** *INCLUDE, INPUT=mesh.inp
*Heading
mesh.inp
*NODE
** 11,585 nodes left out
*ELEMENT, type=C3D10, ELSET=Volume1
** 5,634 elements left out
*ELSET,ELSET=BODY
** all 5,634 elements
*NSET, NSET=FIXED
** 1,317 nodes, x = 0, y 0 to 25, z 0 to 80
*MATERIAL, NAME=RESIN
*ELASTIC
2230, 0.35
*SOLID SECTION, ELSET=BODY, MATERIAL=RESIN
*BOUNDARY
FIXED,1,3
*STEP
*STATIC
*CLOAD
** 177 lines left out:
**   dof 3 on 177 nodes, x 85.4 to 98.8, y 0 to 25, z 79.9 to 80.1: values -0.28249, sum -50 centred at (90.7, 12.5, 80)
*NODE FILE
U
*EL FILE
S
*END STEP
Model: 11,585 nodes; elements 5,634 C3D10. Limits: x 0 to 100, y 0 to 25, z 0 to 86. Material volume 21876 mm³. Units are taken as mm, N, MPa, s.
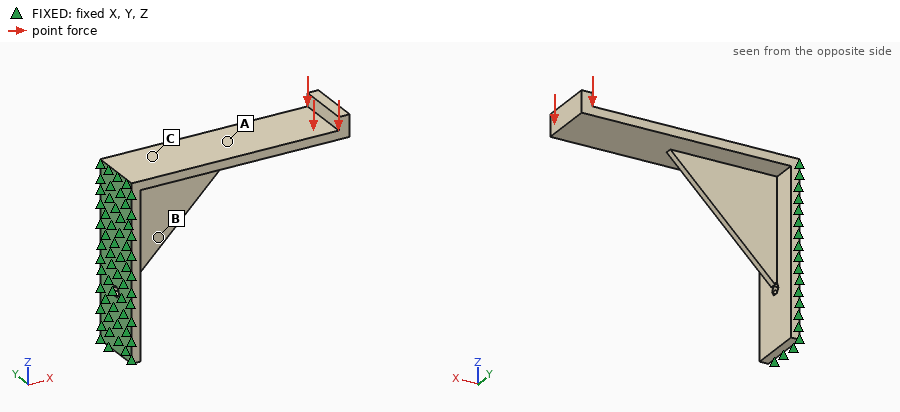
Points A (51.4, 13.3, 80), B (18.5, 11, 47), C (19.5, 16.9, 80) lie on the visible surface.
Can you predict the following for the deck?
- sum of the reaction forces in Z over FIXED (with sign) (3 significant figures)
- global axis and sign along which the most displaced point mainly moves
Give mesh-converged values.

50.0 N
-Z
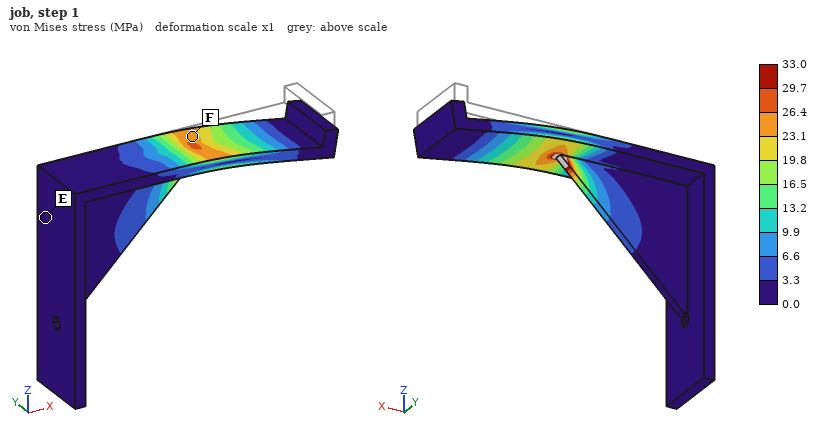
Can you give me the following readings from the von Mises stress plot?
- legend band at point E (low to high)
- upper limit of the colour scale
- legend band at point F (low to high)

0.0 to 3.3 MPa
33.0 MPa
23.1 to 26.4 MPa
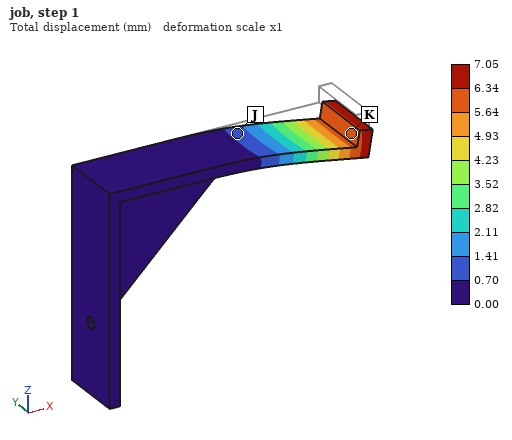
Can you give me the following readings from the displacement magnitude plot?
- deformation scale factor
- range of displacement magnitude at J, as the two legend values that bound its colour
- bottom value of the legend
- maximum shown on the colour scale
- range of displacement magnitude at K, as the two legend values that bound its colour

1
0.70 to 1.41 mm
0.00 mm
7.05 mm
5.64 to 6.34 mm
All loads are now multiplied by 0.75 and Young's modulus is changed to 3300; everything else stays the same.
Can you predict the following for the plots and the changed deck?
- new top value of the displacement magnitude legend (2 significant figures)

3.6 mm
